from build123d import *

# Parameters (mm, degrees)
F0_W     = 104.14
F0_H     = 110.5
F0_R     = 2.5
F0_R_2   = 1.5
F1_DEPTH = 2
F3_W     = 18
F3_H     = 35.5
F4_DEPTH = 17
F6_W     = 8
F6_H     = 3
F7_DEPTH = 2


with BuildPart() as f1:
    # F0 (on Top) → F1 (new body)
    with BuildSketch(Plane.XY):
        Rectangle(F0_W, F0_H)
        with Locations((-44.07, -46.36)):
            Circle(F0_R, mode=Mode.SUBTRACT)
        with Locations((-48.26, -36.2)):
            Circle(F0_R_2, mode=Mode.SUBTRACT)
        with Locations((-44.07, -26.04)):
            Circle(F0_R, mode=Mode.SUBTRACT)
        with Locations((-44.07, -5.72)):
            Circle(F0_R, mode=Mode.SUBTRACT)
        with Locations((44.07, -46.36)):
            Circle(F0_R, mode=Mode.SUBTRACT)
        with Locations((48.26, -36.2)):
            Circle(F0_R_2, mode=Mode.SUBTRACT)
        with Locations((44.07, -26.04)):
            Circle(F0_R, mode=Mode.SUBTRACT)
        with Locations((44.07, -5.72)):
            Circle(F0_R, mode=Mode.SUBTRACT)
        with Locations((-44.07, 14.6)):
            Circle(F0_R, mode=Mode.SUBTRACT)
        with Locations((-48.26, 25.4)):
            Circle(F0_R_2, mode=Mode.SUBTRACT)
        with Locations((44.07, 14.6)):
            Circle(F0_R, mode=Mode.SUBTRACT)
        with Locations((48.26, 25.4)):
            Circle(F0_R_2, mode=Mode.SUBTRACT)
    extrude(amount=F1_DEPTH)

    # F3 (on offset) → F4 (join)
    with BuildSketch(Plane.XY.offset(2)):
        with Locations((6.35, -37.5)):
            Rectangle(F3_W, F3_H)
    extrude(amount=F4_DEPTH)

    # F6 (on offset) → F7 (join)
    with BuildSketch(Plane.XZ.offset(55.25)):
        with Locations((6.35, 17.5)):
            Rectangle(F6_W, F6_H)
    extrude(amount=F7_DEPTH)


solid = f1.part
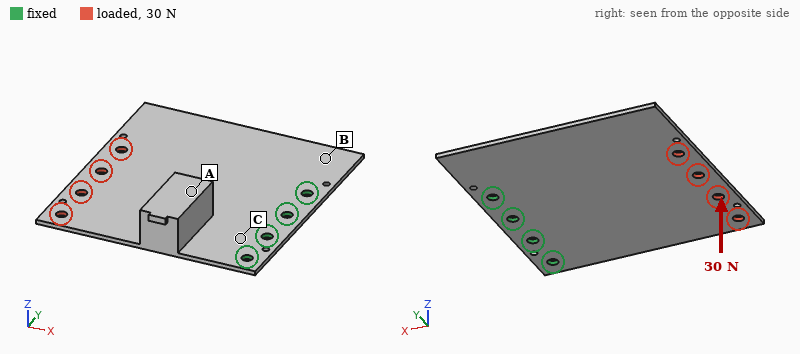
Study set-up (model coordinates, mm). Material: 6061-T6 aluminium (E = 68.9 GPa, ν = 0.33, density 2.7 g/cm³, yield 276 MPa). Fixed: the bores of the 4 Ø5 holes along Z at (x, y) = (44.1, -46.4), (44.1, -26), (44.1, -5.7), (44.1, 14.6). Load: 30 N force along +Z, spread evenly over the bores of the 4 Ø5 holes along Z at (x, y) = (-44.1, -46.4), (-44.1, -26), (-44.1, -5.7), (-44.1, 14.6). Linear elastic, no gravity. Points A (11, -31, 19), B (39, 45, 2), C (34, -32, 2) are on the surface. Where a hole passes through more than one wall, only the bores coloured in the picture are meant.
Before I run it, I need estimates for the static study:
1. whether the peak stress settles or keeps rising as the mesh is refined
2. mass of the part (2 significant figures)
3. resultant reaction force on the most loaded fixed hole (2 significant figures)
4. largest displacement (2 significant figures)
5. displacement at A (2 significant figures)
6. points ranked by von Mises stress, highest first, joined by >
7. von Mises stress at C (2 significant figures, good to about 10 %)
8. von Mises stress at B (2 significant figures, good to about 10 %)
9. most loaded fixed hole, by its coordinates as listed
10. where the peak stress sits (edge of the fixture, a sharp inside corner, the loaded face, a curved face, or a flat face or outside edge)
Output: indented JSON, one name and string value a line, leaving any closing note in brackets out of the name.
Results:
{
  "whether the peak stress settles or keeps rising as the mesh is refined": "keeps rising",
  "mass of the part": "91 g",
  "resultant reaction force on the most loaded fixed hole": "13 N",
  "largest displacement": "1.4 mm",
  "displacement at A": "0.37 mm",
  "points ranked by von Mises stress, highest first, joined by >": "C > B > A",
  "von Mises stress at C": "36 MPa",
  "von Mises stress at B": "11 MPa",
  "most loaded fixed hole, by its coordinates as listed": "(44.1, -5.7)",
  "where the peak stress sits": "edge of the fixture"
}
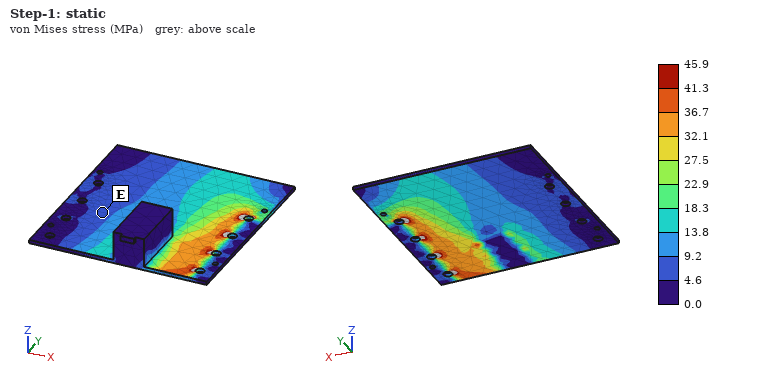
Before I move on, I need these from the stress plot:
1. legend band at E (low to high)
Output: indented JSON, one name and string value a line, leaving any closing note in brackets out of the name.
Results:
{
  "legend band at E": "4.6 to 9.2 MPa"
}
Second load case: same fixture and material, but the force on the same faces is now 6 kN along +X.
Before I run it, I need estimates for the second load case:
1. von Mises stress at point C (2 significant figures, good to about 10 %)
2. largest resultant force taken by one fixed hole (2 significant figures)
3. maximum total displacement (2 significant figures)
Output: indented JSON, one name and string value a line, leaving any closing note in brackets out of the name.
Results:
{
  "von Mises stress at point C": "35 MPa",
  "largest resultant force taken by one fixed hole": "1.7 kN",
  "maximum total displacement": "84 µm"
}
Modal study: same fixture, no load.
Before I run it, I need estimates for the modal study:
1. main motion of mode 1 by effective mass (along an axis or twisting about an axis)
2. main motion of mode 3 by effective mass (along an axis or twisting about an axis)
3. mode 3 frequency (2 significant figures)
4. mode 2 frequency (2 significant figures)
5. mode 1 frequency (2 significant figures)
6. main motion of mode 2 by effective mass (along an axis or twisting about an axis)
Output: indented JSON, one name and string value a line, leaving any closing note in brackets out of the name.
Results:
{
  "main motion of mode 1 by effective mass": "along Z",
  "main motion of mode 3 by effective mass": "along Z",
  "mode 3 frequency": "800 Hz",
  "mode 2 frequency": "360 Hz",
  "mode 1 frequency": "170 Hz",
  "main motion of mode 2 by effective mass": "twisting about X"
}
